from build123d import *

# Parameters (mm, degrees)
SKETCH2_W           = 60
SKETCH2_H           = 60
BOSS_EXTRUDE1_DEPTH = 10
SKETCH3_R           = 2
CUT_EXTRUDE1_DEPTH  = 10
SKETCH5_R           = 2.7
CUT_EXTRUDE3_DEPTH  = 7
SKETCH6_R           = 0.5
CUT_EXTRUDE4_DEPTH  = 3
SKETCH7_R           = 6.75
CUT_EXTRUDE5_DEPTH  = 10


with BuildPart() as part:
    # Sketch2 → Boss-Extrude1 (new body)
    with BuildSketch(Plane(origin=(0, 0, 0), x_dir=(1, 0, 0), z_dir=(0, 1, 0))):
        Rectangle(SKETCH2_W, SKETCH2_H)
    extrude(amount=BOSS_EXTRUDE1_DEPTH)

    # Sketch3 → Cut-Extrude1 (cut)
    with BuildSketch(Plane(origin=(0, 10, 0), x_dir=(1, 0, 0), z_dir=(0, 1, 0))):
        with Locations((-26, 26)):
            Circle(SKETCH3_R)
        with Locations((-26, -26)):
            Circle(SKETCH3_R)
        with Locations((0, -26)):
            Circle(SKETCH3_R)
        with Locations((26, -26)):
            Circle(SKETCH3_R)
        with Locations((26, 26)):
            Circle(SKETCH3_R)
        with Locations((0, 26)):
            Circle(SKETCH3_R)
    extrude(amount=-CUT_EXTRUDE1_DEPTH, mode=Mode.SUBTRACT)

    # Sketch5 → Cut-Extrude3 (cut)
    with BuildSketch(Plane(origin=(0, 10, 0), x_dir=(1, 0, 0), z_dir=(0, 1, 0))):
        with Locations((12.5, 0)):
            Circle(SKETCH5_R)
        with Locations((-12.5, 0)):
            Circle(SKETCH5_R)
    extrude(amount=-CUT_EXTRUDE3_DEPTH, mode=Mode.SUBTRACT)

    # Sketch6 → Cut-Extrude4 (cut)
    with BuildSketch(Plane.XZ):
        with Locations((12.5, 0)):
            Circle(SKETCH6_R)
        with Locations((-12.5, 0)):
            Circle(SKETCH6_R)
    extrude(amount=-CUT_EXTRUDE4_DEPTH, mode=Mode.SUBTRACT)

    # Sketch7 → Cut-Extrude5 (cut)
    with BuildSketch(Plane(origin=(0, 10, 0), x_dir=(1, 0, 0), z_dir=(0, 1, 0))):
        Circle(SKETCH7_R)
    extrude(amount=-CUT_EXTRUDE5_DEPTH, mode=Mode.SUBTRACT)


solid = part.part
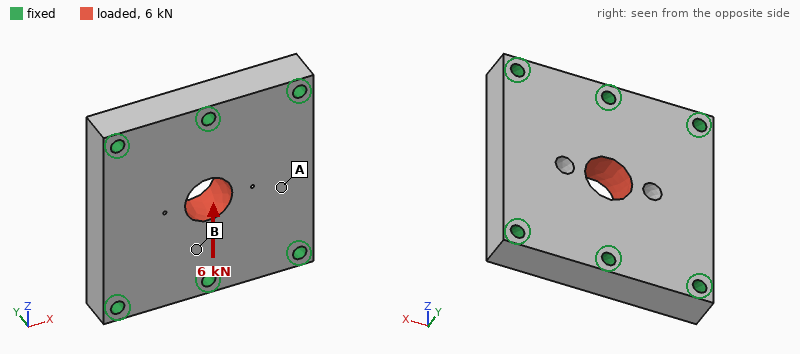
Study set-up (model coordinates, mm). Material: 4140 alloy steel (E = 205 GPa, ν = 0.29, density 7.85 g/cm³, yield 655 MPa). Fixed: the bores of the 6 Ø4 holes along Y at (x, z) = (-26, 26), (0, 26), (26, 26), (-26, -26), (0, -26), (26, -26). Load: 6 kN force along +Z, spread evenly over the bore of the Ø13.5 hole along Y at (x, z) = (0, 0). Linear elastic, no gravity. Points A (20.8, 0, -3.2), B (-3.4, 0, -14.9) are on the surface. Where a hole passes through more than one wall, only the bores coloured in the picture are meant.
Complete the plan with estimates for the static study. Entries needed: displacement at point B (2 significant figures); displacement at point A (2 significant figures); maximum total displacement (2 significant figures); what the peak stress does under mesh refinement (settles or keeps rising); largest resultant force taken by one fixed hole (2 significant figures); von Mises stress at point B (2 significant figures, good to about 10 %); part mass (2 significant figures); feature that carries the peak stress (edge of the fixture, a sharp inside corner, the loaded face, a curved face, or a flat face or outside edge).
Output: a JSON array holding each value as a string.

["0.74 µm", "0.38 µm", "1.4 µm", "keeps rising", "1.7 kN", "12 MPa", "260 g", "edge of the fixture"]
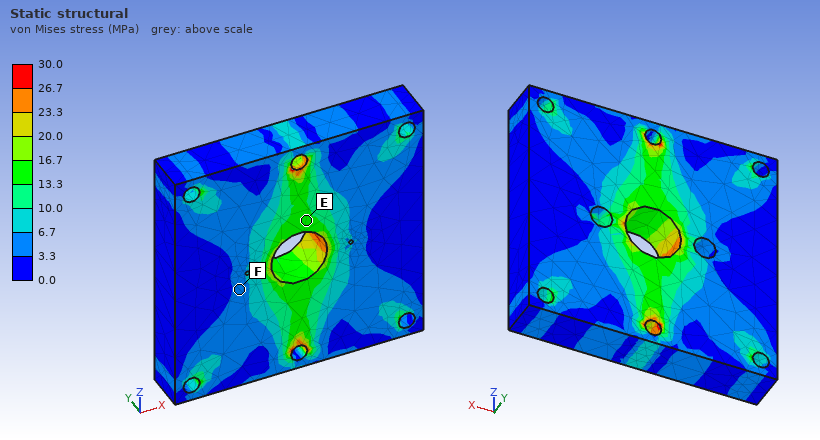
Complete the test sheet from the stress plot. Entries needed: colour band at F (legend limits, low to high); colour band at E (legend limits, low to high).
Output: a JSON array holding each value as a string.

["3.3 to 6.7 MPa", "13.3 to 16.7 MPa"]
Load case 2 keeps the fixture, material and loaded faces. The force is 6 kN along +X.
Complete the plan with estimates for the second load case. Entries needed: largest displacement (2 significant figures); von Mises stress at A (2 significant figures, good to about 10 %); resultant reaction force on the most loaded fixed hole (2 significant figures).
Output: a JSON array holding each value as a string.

["2.4 µm", "4.8 MPa", "1.3 kN"]
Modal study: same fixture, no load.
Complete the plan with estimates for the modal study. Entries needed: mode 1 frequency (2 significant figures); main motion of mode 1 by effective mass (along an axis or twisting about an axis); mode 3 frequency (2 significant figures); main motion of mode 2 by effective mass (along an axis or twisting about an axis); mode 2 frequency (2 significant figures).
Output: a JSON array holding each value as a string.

["14 kHz", "along Y", "26 kHz", "twisting about Z", "17 kHz"]
